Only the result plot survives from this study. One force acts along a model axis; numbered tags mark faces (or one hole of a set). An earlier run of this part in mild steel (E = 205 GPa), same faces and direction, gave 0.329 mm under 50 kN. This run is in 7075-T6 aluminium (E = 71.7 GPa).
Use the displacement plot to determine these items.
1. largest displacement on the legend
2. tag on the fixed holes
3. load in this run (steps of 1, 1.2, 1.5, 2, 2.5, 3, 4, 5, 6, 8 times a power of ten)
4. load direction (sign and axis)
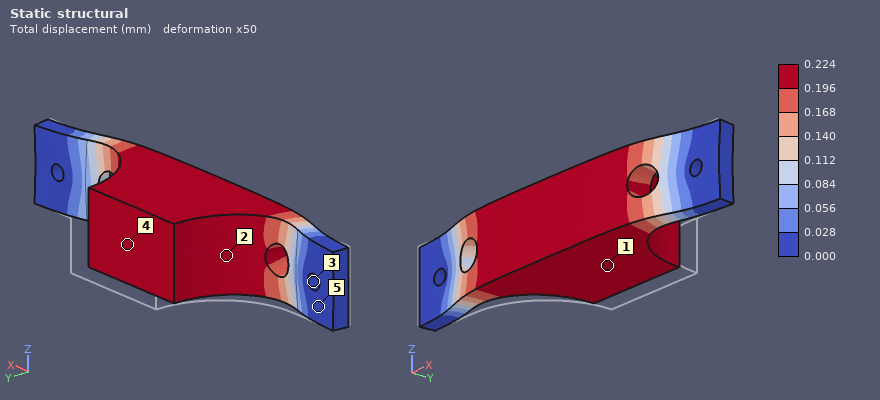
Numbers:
0.224 mm
3
12 kN
-Y
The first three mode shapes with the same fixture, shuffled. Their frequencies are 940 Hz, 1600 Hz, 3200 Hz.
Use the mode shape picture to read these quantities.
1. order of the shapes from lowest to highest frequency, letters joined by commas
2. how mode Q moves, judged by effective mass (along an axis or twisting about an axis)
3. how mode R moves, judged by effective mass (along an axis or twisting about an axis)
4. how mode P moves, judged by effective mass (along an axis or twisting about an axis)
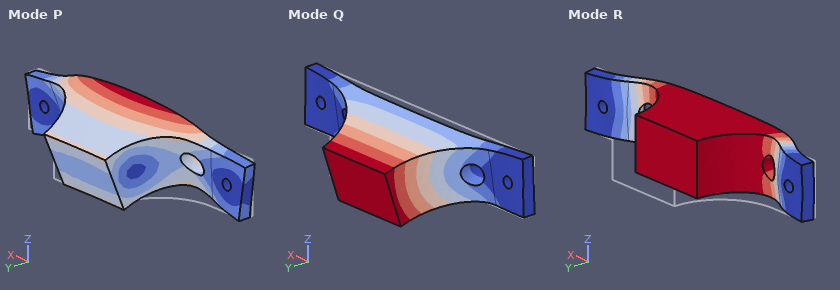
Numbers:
Q, R, P
along Z
along Y
along Z
